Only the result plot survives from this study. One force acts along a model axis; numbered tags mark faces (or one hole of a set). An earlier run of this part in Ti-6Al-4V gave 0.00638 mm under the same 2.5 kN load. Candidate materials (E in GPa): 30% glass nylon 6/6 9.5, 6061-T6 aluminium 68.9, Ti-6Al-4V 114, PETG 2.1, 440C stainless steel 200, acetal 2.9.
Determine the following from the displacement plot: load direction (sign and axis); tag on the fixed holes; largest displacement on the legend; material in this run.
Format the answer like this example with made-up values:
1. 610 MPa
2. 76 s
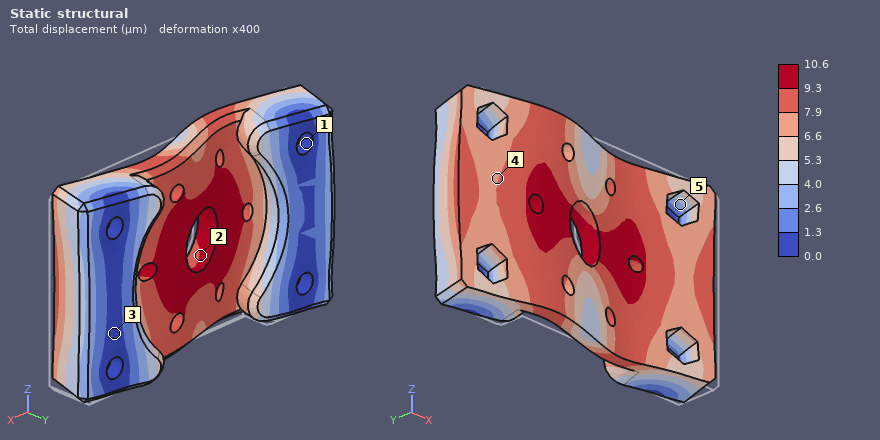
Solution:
1. -X
2. 1
3. 10.6 µm
4. 6061-T6 aluminium
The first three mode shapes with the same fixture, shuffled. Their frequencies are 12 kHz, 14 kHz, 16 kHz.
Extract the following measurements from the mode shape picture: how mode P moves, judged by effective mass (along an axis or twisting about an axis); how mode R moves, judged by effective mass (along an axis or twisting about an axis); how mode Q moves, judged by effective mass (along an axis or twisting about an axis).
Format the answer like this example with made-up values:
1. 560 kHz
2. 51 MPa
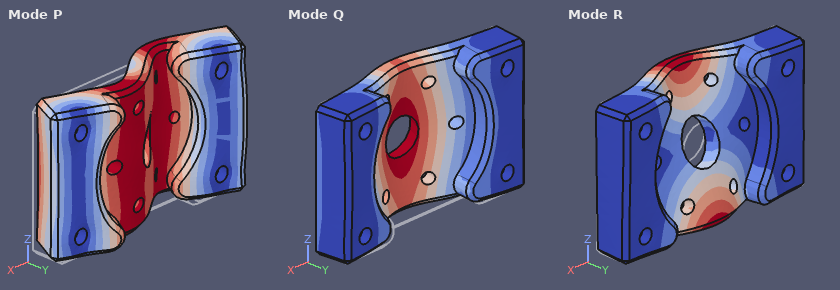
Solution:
1. along X
2. twisting about X
3. along Y
